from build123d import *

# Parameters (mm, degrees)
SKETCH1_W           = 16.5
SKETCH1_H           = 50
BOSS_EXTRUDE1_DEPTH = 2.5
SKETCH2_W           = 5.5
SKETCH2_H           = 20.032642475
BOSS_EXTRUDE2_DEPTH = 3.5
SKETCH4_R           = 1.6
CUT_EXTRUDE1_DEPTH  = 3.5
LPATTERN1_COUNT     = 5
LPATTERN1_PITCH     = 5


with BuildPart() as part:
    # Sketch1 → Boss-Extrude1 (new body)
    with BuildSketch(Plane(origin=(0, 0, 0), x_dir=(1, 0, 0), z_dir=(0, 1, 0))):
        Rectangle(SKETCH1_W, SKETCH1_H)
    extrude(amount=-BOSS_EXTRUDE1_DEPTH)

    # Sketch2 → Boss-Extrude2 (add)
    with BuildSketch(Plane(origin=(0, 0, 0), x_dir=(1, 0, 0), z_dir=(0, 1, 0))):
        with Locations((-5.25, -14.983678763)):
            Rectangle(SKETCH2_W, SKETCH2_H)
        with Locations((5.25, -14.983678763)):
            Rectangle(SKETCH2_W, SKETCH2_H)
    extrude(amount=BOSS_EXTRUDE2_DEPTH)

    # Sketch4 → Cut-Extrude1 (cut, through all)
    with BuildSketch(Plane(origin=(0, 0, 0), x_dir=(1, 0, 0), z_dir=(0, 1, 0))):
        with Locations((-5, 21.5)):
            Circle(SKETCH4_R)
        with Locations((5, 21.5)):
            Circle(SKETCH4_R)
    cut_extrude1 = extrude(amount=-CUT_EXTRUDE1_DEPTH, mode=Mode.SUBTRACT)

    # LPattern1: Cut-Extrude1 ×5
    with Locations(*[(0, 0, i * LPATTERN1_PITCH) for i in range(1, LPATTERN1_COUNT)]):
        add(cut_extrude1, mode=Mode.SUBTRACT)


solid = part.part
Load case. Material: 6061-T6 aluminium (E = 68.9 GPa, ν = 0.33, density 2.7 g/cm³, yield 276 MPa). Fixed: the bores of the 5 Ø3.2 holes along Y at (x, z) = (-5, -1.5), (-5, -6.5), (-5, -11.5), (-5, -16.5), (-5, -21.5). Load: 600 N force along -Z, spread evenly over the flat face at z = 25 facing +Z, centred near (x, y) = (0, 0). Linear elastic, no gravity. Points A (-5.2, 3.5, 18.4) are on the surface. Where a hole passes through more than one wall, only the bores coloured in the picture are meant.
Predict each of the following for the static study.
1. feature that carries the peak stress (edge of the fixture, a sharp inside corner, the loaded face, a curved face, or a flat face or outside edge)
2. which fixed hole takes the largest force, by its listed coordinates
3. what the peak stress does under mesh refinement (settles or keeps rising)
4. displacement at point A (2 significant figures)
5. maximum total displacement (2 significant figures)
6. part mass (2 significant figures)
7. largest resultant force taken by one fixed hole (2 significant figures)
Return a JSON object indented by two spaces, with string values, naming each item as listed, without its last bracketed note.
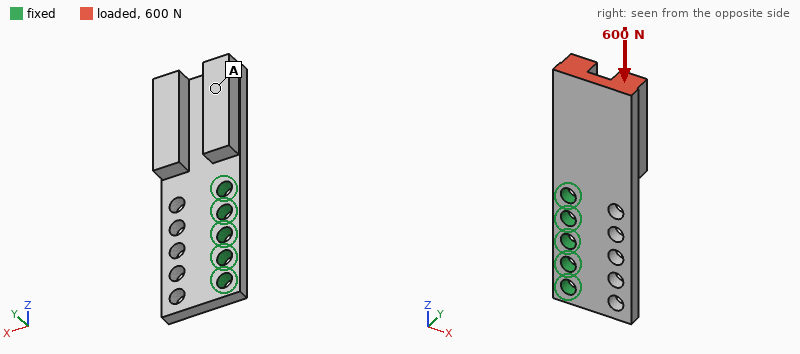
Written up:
{
  "feature that carries the peak stress": "edge of the fixture",
  "which fixed hole takes the largest force, by its listed coordinates": "(-5, -1.5)",
  "what the peak stress does under mesh refinement": "keeps rising",
  "displacement at point A": "0.080 mm",
  "maximum total displacement": "0.12 mm",
  "part mass": "7.1 g",
  "largest resultant force taken by one fixed hole": "370 N"
}
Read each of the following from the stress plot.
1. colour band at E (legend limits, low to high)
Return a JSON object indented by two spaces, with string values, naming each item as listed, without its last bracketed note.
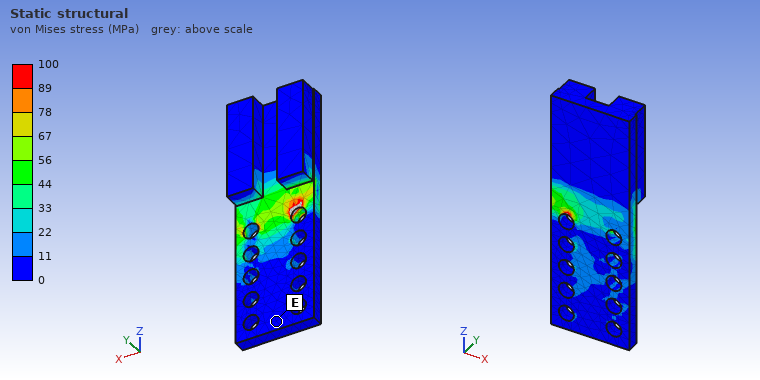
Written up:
{
  "colour band at E": "0 to 11 MPa"
}
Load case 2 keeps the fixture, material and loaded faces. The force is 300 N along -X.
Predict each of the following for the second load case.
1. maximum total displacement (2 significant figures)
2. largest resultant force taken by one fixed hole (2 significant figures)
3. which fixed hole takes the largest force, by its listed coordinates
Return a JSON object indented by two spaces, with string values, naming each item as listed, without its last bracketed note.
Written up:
{
  "maximum total displacement": "75 µm",
  "largest resultant force taken by one fixed hole": "840 N",
  "which fixed hole takes the largest force, by its listed coordinates": "(-5, -1.5)"
}
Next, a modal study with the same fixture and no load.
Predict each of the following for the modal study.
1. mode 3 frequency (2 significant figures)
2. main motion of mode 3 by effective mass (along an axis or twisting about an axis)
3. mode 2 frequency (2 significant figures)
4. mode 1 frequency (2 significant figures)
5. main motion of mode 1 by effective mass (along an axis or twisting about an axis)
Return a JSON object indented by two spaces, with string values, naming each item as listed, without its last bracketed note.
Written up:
{
  "mode 3 frequency": "8300 Hz",
  "main motion of mode 3 by effective mass": "along X",
  "mode 2 frequency": "6400 Hz",
  "mode 1 frequency": "2100 Hz",
  "main motion of mode 1 by effective mass": "along Y"
}
